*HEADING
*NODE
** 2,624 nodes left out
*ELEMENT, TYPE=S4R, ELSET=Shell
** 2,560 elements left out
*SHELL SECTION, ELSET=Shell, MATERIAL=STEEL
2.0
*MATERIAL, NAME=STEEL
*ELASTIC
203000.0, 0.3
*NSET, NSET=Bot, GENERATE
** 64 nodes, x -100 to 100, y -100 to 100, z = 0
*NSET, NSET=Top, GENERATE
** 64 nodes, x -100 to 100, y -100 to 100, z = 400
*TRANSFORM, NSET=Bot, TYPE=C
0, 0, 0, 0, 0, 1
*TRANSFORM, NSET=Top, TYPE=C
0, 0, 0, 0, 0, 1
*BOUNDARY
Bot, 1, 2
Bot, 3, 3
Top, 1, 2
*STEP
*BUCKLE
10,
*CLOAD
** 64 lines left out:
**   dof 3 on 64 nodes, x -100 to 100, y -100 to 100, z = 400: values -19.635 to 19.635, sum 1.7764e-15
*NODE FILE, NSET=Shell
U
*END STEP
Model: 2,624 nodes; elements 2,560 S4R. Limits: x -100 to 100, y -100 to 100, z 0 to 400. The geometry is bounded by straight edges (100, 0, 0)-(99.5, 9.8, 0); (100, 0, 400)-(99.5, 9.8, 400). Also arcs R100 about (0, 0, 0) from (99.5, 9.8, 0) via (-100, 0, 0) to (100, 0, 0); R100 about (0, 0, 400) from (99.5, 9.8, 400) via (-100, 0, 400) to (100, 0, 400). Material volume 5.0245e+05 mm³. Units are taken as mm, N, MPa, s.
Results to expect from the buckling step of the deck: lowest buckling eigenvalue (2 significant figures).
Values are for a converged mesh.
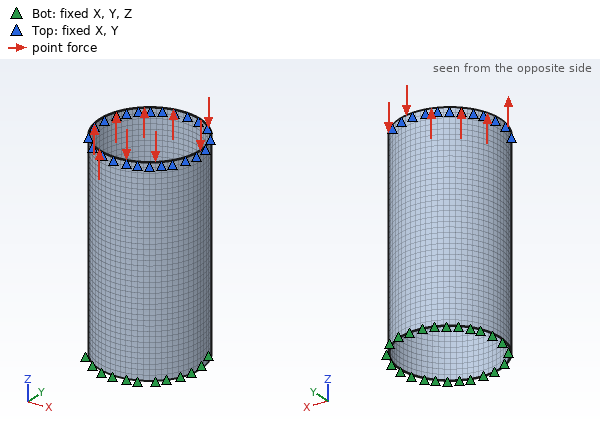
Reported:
2700
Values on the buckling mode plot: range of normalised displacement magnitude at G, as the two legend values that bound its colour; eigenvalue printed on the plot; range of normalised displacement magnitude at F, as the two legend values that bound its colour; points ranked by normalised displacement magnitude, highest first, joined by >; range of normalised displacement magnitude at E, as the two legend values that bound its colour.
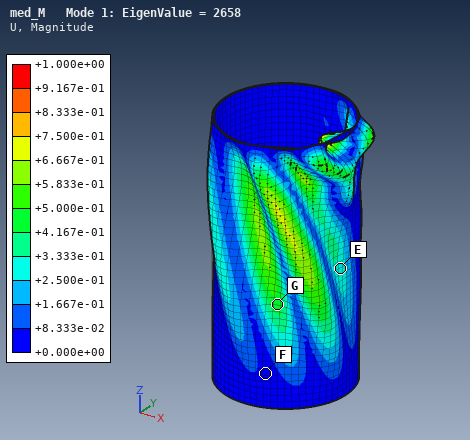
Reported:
+4.167e-01 to +5.000e-01
2658
+0.000e+00 to +8.333e-02
G > E > F
+2.500e-01 to +3.333e-01
